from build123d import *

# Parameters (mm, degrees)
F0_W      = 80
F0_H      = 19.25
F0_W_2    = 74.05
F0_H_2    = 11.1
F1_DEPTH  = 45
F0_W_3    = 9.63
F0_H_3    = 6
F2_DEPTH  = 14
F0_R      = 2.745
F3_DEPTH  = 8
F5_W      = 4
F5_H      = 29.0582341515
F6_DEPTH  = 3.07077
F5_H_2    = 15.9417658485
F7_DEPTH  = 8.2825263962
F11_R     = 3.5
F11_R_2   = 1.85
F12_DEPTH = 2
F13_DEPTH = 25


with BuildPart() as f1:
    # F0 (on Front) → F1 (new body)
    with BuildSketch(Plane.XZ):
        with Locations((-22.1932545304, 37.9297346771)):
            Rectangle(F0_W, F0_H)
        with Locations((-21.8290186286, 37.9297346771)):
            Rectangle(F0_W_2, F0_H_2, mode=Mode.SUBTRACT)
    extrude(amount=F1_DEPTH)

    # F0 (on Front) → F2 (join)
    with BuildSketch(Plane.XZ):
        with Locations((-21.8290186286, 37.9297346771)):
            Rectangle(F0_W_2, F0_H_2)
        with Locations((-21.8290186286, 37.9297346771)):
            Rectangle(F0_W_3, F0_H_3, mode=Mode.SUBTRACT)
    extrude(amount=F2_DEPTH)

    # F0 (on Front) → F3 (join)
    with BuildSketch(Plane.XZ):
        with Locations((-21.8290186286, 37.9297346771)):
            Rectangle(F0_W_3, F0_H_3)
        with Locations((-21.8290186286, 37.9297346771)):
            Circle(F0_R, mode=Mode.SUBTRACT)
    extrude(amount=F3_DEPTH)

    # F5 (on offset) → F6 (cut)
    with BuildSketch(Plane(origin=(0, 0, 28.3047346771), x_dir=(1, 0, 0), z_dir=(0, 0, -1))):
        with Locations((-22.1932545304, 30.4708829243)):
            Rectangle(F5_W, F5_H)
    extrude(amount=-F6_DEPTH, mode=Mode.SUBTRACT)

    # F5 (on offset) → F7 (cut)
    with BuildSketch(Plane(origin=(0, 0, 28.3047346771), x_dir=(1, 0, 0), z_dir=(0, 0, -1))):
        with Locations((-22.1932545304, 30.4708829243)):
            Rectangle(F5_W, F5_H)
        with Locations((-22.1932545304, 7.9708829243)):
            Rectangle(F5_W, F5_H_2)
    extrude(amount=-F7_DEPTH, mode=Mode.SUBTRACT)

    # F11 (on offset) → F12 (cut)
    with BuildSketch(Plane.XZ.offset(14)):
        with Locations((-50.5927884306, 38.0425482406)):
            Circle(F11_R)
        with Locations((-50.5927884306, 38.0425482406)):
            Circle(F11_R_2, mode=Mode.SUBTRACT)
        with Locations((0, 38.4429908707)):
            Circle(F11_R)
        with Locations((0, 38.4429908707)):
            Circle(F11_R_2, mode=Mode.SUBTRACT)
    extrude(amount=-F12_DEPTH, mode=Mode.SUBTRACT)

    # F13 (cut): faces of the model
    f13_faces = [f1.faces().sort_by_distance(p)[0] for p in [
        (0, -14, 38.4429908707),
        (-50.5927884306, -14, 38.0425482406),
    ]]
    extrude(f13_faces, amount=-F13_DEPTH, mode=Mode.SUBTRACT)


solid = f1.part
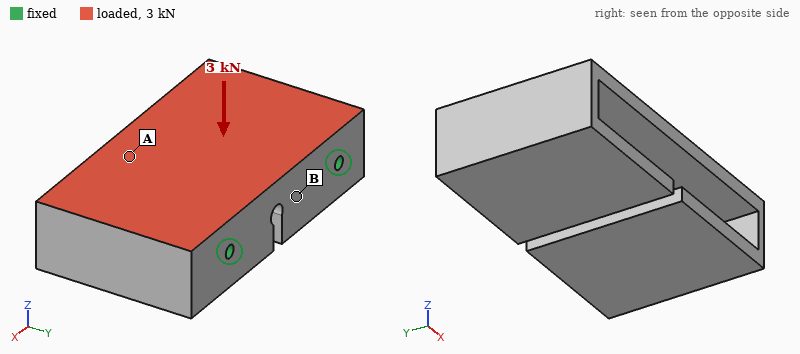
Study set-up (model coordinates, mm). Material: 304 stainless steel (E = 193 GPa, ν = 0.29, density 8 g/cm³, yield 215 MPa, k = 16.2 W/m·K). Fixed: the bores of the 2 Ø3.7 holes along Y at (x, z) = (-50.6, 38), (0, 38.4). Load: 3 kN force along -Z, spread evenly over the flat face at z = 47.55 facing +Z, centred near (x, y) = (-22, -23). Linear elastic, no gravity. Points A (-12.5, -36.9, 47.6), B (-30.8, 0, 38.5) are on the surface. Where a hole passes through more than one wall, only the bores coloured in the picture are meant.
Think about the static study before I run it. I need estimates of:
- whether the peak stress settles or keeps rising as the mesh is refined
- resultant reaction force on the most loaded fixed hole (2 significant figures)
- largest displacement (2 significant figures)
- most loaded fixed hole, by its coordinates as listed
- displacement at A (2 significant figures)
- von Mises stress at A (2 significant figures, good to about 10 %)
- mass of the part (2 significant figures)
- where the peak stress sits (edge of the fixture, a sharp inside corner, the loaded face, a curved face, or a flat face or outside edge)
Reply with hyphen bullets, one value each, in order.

- keeps rising
- 1.8 kN
- 69 µm
- (0, 38.4)
- 48 µm
- 27 MPa
- 340 g
- edge of the fixture
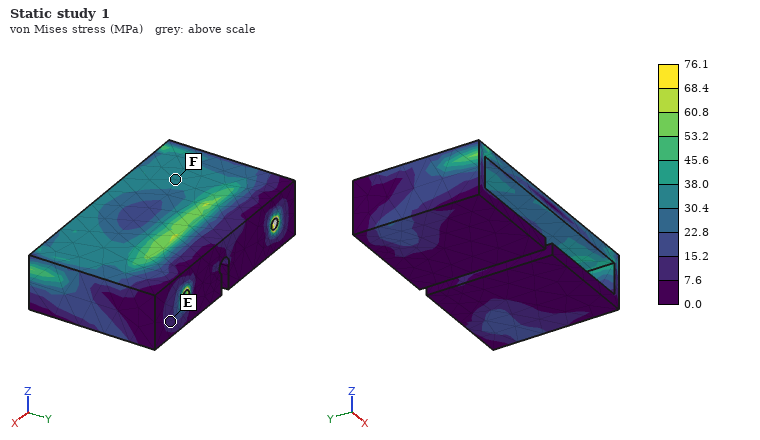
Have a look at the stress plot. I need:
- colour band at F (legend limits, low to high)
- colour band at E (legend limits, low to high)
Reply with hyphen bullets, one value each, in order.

- 30.4 to 38.0 MPa
- 7.6 to 15.2 MPa
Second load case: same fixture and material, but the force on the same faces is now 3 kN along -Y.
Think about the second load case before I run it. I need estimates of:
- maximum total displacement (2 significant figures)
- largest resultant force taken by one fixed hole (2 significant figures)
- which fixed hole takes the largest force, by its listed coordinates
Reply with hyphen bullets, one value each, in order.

- 18 µm
- 1.7 kN
- (0, 38.4)
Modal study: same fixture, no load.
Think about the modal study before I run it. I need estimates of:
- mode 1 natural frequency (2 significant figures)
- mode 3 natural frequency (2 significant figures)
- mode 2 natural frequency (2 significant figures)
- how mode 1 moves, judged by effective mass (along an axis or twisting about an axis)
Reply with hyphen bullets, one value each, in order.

- 3700 Hz
- 4700 Hz
- 4100 Hz
- along Z
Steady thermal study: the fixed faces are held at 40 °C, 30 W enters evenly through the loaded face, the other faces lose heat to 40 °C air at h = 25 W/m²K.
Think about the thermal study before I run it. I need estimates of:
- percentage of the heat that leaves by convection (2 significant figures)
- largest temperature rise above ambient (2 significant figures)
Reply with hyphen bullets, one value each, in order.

- 28 %
- 68 K
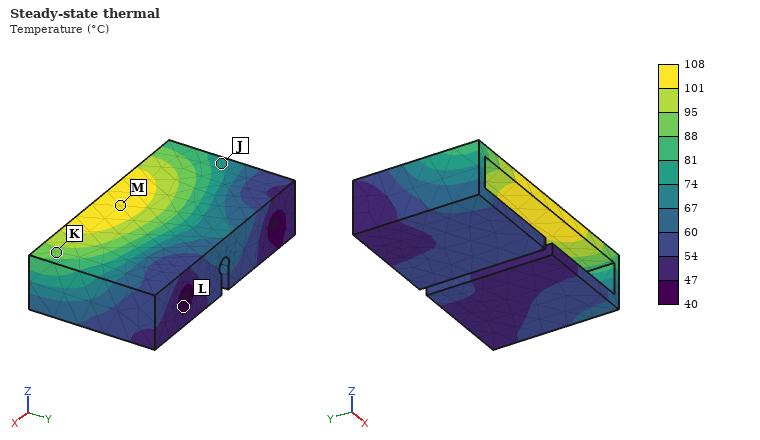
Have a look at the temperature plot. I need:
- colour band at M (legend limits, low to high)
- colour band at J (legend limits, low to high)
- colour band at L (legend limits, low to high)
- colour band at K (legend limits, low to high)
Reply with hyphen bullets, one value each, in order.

- 101 to 108 °C
- 74 to 81 °C
- 40 to 47 °C
- 88 to 95 °C
